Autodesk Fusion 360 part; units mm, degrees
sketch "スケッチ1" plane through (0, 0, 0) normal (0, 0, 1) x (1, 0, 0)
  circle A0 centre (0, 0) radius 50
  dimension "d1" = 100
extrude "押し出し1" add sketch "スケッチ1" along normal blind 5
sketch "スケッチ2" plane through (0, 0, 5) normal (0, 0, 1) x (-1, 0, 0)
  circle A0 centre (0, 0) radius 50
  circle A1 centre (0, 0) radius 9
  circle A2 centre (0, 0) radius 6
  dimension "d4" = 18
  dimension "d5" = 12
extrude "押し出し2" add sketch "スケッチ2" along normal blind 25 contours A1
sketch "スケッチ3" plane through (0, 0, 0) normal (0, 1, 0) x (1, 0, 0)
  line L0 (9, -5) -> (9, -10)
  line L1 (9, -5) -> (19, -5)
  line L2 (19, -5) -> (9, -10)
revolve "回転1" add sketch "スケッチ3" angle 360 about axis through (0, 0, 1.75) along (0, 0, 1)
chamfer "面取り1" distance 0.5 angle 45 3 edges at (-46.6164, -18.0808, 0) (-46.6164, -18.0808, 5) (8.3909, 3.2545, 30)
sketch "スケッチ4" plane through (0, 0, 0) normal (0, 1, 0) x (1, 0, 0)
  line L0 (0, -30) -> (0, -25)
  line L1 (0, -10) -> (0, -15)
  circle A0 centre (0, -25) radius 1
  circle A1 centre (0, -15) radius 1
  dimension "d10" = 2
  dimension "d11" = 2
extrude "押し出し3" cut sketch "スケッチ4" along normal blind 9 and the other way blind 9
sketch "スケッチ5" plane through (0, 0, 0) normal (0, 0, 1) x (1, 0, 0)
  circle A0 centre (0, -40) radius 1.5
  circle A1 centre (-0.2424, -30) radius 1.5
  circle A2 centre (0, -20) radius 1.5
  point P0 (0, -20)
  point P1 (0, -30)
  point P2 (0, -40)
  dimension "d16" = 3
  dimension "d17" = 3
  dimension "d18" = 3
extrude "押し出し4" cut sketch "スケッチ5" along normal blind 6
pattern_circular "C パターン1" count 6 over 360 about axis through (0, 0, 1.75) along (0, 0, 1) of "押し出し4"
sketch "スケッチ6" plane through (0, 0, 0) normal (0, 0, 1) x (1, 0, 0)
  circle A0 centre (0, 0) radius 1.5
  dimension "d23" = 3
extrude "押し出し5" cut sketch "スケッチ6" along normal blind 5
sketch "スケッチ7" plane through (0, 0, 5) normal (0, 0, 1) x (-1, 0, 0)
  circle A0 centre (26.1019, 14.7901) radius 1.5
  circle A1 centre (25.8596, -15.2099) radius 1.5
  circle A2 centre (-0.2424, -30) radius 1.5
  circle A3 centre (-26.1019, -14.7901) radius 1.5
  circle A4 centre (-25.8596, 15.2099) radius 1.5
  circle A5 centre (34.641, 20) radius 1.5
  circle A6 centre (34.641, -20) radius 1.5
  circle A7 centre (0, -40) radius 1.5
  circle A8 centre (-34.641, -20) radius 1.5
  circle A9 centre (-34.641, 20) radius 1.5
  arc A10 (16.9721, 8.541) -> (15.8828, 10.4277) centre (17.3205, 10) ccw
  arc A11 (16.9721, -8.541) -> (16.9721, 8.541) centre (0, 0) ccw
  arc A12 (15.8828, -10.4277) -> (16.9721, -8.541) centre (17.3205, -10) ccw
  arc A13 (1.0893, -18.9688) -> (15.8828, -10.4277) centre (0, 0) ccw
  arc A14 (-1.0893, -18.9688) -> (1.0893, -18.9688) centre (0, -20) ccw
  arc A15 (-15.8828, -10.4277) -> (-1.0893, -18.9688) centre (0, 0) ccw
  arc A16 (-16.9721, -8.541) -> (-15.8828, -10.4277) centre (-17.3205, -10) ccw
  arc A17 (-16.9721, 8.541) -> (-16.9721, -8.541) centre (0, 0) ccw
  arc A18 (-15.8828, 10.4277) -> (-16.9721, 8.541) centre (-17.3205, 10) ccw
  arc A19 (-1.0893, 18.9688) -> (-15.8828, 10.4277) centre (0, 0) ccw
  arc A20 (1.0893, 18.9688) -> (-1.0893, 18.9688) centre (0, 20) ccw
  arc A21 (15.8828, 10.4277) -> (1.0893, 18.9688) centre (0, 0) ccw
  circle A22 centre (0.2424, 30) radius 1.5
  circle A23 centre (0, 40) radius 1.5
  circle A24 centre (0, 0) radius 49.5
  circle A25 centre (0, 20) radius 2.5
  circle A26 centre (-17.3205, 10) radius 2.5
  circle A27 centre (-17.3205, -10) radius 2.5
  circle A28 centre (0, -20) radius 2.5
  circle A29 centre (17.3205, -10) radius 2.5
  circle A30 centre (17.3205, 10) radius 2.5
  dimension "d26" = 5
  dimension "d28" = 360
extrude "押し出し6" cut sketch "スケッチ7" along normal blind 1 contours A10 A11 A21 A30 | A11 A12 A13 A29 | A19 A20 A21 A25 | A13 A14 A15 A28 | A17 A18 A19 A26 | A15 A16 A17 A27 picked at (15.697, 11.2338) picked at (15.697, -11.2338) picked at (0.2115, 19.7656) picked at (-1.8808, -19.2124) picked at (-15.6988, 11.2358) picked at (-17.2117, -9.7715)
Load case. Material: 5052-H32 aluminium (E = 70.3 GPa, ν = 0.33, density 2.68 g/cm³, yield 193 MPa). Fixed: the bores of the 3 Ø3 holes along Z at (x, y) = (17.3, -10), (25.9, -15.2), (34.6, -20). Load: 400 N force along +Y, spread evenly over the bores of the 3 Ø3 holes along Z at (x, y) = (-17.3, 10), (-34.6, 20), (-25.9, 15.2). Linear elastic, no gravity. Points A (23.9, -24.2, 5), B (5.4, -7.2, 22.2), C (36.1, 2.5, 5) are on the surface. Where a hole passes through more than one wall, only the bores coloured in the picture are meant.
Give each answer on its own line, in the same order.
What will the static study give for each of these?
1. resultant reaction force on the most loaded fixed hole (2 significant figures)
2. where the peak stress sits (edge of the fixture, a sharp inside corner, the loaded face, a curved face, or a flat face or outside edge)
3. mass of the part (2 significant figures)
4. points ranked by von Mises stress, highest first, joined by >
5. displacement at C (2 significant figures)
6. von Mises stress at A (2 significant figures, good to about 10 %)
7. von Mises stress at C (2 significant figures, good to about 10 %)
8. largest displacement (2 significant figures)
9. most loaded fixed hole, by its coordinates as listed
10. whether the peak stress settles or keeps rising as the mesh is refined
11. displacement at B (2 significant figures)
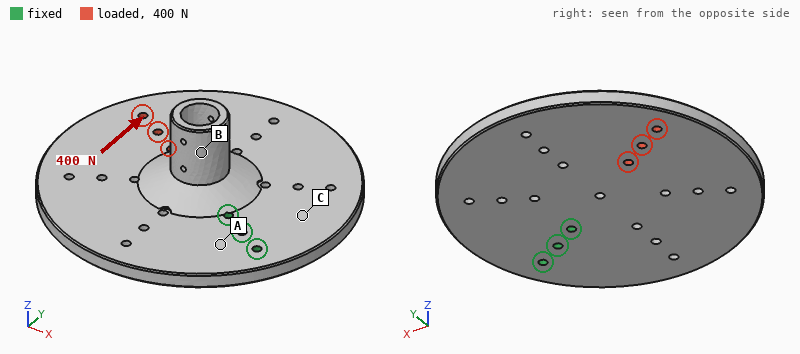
1.1 kN
edge of the fixture
120 g
A > C > B
4.0 µm
6.7 MPa
3.4 MPa
21 µm
(17.3, -10)
keeps rising
3.4 µm
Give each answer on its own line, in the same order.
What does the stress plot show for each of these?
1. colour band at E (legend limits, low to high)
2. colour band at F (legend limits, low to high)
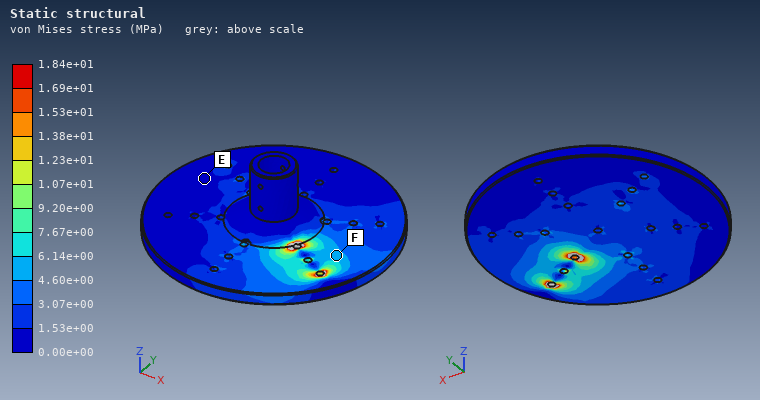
0.00e+00 to 1.53e+00 MPa
4.60e+00 to 6.14e+00 MPa
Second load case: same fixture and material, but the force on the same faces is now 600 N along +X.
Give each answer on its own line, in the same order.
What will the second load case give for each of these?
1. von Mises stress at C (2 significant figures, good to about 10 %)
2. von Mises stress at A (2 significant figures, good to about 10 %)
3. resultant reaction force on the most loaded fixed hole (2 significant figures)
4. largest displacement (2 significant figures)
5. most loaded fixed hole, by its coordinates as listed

3.8 MPa
4.1 MPa
1.0 kN
19 µm
(17.3, -10)
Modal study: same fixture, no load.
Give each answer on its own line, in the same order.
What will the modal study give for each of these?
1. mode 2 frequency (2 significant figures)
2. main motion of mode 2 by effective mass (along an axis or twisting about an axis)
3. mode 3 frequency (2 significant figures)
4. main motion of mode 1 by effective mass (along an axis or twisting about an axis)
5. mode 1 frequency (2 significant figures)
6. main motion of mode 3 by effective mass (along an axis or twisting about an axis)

1300 Hz
twisting about X
2900 Hz
along Z
950 Hz
along Z
